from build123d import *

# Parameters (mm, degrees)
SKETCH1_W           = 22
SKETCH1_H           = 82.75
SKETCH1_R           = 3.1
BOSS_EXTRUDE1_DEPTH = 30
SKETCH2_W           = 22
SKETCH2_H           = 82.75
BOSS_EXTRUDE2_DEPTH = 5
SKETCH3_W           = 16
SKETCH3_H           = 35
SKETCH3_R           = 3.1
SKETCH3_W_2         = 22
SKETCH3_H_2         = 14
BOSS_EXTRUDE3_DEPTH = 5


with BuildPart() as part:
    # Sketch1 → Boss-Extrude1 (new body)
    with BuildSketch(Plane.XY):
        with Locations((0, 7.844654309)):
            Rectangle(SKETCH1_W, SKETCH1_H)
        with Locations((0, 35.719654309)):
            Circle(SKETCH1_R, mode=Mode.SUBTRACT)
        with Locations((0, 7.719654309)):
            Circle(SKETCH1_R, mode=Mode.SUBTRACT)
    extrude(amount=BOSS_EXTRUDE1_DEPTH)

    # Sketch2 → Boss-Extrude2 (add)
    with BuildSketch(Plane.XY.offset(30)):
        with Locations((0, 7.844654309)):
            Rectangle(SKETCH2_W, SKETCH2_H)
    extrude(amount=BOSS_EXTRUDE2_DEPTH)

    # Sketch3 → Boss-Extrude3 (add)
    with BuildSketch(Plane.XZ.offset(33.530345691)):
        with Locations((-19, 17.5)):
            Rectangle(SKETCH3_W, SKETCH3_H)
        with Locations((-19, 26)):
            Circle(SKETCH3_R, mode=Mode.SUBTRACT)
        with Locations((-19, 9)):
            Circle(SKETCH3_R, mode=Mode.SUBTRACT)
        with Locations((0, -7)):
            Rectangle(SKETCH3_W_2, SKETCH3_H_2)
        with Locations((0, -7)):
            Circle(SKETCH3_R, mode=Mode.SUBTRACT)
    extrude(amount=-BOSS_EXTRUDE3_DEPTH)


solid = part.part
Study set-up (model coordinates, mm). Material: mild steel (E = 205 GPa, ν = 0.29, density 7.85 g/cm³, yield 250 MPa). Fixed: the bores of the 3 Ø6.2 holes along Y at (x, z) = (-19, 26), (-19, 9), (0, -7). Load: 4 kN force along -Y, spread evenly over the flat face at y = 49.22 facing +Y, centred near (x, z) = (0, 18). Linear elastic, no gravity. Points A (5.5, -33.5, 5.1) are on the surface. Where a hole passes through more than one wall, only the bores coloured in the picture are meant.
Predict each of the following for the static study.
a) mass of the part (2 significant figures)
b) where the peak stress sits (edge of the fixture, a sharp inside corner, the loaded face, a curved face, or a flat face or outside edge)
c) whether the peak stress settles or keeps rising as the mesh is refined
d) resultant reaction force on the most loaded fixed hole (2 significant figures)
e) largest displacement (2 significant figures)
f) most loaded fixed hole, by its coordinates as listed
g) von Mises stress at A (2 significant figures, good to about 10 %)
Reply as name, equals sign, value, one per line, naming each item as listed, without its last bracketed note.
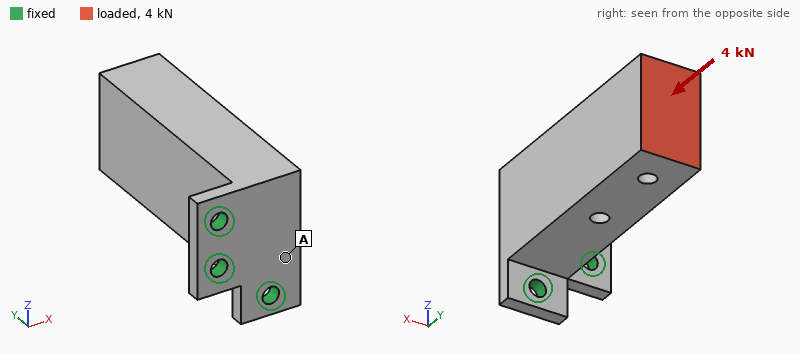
mass of the part = 520 g
where the peak stress sits = edge of the fixture
whether the peak stress settles or keeps rising as the mesh is refined = keeps rising
resultant reaction force on the most loaded fixed hole = 2.7 kN
largest displacement = 0.12 mm
most loaded fixed hole, by its coordinates as listed = (-19, 26)
von Mises stress at A = 35 MPa
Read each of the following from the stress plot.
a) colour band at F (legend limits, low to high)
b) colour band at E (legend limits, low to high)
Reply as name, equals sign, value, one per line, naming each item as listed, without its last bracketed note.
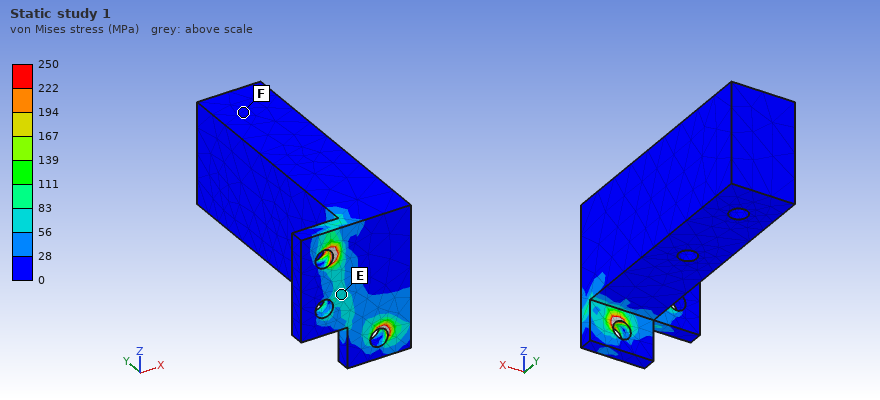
colour band at F = 0 to 28 MPa
colour band at E = 56 to 83 MPa
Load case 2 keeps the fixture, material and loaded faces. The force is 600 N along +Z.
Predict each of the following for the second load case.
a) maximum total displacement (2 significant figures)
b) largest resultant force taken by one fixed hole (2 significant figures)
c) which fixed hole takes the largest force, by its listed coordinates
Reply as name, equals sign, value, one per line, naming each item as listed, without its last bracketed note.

maximum total displacement = 68 µm
largest resultant force taken by one fixed hole = 1.8 kN
which fixed hole takes the largest force, by its listed coordinates = (-19, 26)
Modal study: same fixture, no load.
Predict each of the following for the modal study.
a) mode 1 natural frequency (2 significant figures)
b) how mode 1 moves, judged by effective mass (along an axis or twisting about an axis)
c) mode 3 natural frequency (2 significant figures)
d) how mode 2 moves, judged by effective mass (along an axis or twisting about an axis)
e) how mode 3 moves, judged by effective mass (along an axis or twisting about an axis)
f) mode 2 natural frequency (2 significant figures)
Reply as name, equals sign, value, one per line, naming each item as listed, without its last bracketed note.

mode 1 natural frequency = 820 Hz
how mode 1 moves, judged by effective mass = along X
mode 3 natural frequency = 6400 Hz
how mode 2 moves, judged by effective mass = along Z
how mode 3 moves, judged by effective mass = along Y
mode 2 natural frequency = 1900 Hz
